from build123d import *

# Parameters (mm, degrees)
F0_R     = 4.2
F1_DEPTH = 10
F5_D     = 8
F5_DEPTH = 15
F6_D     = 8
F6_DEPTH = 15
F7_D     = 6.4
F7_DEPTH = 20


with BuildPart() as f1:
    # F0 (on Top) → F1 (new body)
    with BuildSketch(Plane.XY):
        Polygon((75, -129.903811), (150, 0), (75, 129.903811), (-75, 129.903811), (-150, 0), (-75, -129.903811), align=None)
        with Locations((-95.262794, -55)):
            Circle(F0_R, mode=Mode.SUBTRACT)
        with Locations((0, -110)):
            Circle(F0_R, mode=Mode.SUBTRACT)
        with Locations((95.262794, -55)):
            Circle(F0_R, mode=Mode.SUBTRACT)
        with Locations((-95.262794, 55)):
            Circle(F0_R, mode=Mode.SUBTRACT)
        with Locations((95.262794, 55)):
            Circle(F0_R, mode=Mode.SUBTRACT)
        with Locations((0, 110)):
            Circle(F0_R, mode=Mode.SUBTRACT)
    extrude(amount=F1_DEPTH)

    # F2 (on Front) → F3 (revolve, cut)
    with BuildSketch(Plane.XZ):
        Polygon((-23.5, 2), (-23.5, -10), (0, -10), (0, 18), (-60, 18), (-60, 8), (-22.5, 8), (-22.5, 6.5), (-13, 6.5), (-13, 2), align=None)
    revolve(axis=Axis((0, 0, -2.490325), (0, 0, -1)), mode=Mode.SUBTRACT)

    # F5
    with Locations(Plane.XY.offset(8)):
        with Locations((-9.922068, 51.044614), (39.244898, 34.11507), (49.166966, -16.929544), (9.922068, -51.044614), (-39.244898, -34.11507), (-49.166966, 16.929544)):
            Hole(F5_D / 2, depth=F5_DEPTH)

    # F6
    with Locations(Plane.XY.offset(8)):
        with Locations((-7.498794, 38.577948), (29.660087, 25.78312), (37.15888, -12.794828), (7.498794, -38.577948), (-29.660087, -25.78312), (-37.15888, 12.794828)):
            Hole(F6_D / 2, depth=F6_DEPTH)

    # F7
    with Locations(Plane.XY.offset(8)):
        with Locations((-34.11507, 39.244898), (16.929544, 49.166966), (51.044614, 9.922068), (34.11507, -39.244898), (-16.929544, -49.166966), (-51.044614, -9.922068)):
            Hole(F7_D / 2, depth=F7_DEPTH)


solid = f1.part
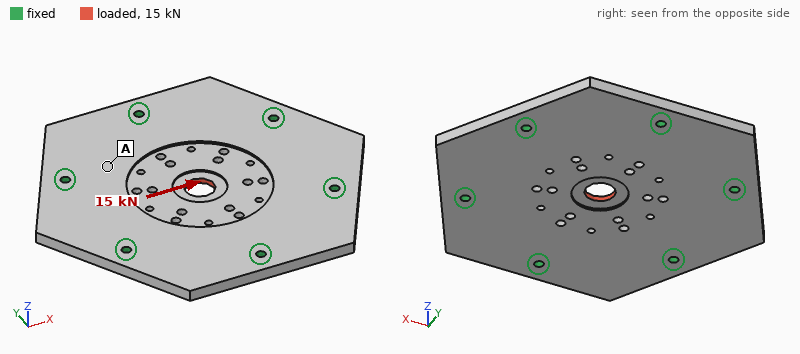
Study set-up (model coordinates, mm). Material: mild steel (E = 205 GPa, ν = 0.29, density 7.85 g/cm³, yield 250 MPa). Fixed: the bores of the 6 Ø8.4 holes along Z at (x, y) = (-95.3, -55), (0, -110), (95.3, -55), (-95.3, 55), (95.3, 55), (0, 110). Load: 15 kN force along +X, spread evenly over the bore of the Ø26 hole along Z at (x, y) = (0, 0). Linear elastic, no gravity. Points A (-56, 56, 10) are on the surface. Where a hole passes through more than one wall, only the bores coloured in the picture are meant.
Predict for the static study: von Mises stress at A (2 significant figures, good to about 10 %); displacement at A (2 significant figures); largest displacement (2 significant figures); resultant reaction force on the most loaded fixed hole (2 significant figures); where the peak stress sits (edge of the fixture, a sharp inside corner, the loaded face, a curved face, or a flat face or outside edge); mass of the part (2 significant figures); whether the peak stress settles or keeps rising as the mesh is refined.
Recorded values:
4.6 MPa
1.2 µm
7.4 µm
3.2 kN
a sharp inside corner
4.3 kg
keeps rising
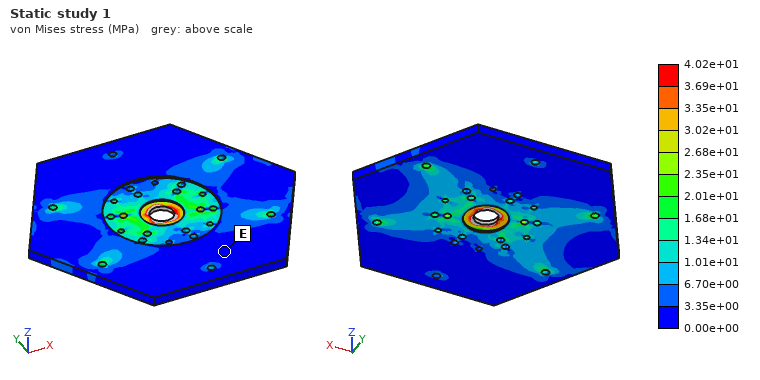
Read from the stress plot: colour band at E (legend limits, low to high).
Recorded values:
0.00e+00 to 3.35e+00 MPa
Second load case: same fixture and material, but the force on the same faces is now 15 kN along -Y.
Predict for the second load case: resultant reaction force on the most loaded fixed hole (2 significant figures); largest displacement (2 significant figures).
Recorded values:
3.7 kN
7.4 µm
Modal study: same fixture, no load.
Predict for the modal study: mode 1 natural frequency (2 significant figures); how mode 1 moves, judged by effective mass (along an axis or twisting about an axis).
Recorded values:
1600 Hz
along Z
